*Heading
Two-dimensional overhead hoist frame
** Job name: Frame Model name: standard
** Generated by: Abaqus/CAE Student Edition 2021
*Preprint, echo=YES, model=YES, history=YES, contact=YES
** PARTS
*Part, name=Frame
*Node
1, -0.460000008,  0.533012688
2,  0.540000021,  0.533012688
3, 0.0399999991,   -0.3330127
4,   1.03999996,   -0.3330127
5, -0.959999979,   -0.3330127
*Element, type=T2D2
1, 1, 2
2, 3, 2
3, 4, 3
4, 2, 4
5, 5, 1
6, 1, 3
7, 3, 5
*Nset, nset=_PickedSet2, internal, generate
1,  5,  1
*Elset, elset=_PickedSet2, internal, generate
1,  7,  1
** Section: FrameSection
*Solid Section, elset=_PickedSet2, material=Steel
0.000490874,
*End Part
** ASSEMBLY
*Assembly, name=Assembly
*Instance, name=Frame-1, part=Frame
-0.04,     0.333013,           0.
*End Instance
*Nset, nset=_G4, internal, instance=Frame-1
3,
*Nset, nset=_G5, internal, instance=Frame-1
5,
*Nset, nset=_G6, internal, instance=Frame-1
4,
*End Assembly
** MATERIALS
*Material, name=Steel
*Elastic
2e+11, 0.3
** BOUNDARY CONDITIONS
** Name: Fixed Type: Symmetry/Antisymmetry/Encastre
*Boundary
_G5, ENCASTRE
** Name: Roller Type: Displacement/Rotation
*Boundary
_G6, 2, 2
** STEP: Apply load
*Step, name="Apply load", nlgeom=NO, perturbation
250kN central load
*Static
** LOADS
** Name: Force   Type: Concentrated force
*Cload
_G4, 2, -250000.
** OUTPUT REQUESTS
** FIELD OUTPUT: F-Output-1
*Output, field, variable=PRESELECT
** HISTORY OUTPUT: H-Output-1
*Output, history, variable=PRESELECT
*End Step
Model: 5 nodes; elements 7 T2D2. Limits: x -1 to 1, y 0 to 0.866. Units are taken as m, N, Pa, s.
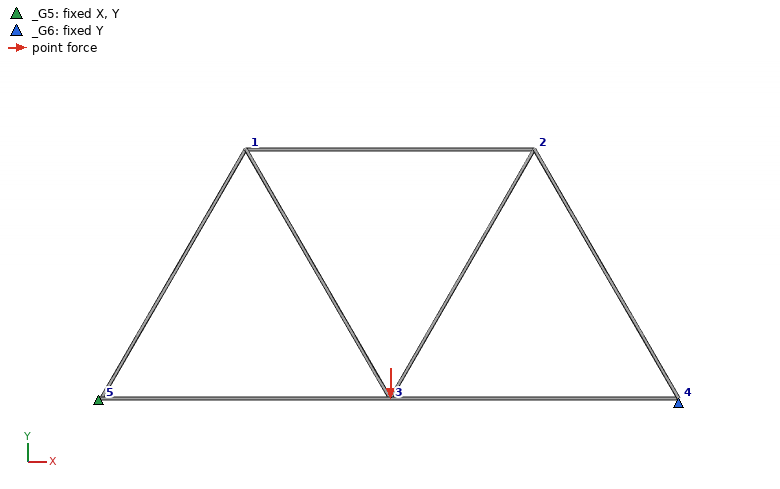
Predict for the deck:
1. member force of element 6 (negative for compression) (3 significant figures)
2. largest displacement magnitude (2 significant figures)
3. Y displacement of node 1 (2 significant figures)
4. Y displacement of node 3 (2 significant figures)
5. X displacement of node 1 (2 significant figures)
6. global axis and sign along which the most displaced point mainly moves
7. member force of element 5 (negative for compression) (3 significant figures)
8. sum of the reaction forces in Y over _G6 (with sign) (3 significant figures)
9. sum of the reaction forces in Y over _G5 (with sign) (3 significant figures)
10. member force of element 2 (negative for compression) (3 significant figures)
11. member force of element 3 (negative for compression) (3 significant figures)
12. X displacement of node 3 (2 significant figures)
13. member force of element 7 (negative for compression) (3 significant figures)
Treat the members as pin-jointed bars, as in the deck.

1.44e+05 N
0.0047 m
-0.0025 m
-0.0047 m
0.0015 m
-Y
-1.44e+05 N
1.25e+05 N
1.25e+05 N
1.44e+05 N
72200 N
7.4e-04 m
72200 N
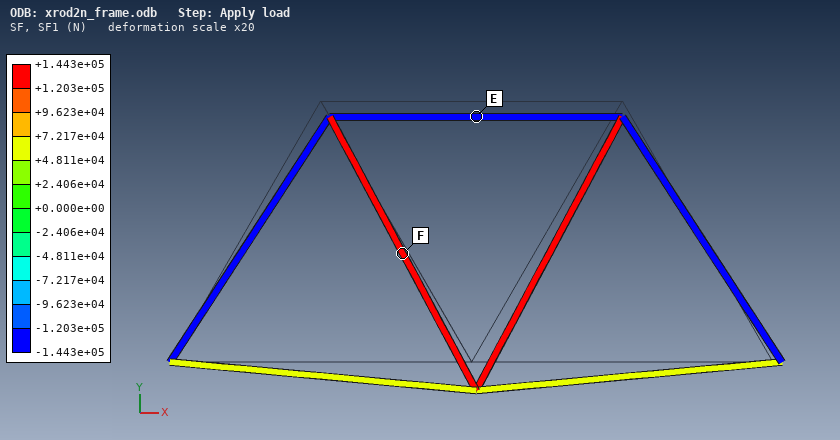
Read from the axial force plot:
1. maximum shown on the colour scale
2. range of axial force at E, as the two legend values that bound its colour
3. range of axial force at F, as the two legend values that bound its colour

+1.443e+05 N
-1.443e+05 to -1.203e+05 N
+1.203e+05 to +1.443e+05 N
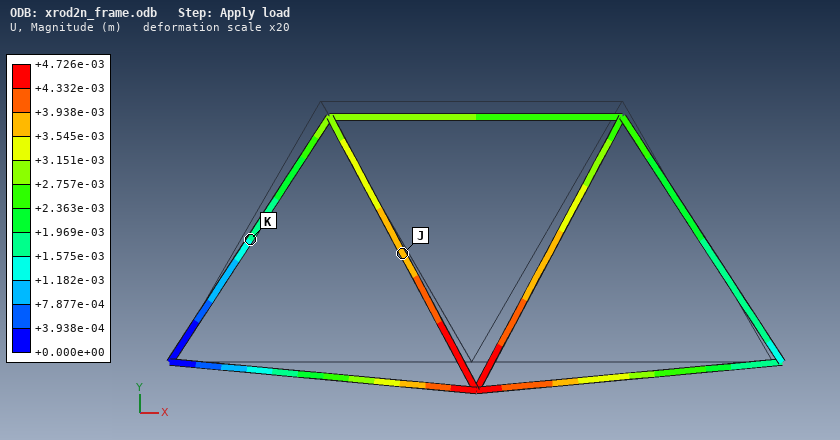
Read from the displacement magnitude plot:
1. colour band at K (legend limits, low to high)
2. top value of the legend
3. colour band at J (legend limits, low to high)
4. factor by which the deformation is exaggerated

+1.182e-03 to +1.575e-03 m
+4.726e-03 m
+3.545e-03 to +3.938e-03 m
20
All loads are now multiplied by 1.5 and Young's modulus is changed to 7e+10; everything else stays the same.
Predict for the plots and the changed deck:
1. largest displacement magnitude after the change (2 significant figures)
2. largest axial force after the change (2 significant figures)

0.020 m
2.2e+05 N
